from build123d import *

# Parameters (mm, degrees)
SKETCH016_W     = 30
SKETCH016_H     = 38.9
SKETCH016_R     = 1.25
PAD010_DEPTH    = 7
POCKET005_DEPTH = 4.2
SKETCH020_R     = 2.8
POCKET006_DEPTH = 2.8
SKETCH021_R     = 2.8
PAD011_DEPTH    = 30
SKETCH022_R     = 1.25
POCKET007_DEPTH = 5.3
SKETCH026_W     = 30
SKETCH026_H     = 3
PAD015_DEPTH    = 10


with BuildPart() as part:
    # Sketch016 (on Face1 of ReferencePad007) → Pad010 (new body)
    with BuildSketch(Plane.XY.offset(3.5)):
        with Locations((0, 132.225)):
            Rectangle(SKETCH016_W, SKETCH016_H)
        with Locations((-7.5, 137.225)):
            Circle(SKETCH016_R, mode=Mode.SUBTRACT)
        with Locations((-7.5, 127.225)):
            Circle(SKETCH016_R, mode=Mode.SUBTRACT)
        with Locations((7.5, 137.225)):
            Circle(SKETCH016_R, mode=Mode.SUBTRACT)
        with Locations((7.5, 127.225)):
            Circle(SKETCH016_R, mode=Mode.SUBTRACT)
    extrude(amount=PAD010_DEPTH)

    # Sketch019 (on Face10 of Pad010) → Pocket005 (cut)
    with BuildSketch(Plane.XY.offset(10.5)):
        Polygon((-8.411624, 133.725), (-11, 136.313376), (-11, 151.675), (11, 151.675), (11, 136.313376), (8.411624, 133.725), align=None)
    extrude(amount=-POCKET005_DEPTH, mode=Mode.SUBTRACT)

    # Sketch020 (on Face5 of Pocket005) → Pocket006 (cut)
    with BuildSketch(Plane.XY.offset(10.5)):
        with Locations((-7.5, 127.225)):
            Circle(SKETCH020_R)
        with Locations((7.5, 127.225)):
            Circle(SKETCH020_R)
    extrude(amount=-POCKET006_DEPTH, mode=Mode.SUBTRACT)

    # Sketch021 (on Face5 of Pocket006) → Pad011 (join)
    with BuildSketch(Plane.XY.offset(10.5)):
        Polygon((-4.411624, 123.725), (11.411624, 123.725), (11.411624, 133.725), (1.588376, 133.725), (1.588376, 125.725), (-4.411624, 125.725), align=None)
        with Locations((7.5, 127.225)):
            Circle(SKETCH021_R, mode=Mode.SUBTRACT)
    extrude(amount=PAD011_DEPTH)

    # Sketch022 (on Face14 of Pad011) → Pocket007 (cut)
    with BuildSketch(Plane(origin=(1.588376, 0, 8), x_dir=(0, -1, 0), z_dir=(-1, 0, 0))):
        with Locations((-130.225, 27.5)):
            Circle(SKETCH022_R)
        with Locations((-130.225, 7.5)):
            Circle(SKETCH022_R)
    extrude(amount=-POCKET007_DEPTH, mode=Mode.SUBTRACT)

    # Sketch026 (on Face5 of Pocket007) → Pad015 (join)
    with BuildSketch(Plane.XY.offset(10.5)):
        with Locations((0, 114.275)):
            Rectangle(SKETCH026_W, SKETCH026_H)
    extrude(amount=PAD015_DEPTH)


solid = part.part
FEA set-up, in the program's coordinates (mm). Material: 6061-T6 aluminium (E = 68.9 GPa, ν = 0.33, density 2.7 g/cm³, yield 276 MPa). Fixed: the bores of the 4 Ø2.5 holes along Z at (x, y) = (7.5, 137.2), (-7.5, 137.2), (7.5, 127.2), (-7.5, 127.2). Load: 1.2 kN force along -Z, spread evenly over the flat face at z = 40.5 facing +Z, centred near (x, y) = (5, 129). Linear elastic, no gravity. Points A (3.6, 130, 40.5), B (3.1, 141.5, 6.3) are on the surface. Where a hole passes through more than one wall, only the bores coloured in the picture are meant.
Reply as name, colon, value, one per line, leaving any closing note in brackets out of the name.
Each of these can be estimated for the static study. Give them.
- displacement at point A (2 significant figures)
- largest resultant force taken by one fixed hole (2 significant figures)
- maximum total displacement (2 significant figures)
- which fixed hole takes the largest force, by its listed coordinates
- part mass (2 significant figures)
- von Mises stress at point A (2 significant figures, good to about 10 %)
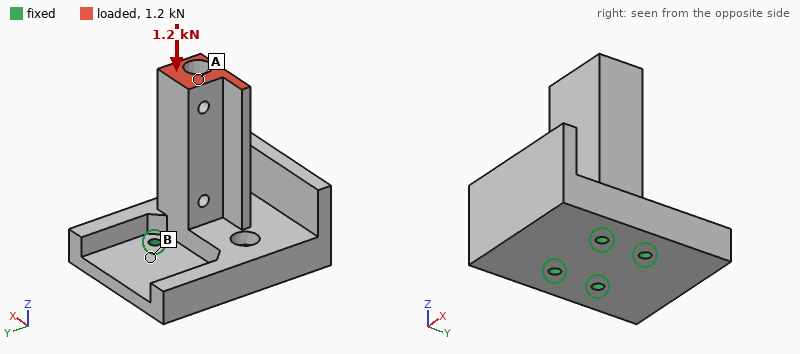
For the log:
displacement at point A: 9.3 µm
largest resultant force taken by one fixed hole: 770 N
maximum total displacement: 9.4 µm
which fixed hole takes the largest force, by its listed coordinates: (7.5, 127.2)
part mass: 26 g
von Mises stress at point A: 11 MPa
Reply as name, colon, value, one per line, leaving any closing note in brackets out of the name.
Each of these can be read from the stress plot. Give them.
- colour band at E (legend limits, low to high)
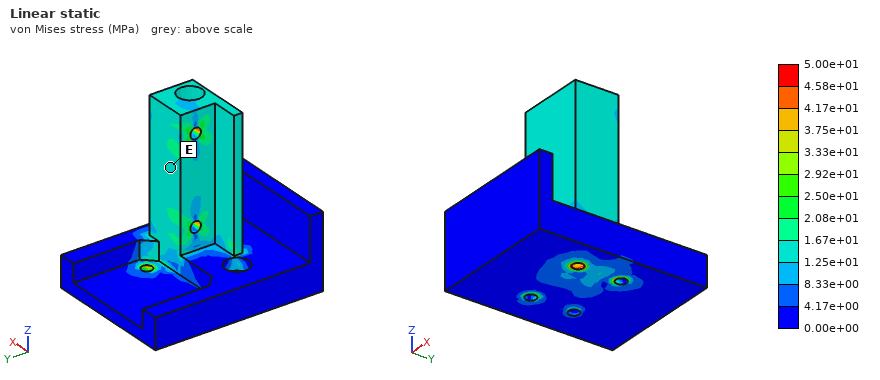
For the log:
colour band at E: 1.25e+01 to 1.67e+01 MPa
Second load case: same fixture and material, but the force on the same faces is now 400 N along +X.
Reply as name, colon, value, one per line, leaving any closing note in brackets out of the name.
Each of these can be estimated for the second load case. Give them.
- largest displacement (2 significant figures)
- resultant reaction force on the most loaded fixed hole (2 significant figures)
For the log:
largest displacement: 90 µm
resultant reaction force on the most loaded fixed hole: 770 N
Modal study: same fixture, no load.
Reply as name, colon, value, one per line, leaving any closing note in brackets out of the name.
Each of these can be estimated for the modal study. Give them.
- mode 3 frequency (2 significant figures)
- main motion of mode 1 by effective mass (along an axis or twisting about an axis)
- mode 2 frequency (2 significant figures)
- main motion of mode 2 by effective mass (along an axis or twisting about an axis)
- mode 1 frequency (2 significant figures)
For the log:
mode 3 frequency: 12 kHz
main motion of mode 1 by effective mass: along Y
mode 2 frequency: 8100 Hz
main motion of mode 2 by effective mass: along X
mode 1 frequency: 5600 Hz
